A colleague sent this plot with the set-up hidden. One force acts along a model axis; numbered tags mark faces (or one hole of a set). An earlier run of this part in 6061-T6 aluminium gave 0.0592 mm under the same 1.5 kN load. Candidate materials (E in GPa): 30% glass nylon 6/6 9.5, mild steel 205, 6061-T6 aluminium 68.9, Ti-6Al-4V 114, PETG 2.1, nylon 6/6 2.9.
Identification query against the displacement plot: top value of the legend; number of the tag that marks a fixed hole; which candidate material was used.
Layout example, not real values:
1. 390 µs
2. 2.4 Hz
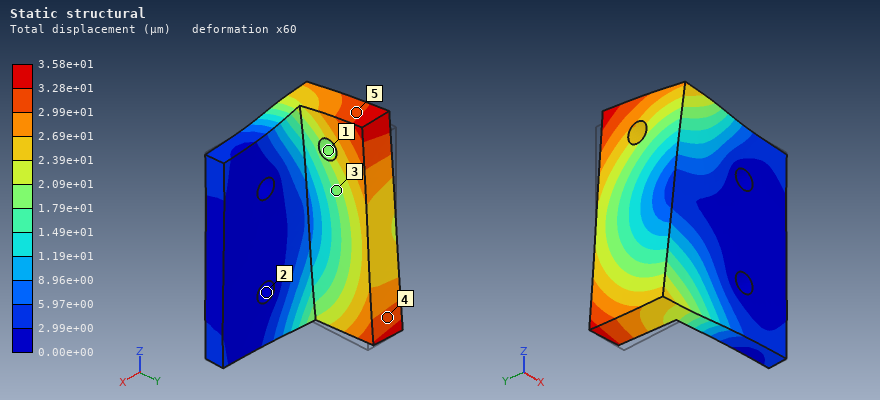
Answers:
1. 3.58e+01 µm
2. 2
3. Ti-6Al-4V
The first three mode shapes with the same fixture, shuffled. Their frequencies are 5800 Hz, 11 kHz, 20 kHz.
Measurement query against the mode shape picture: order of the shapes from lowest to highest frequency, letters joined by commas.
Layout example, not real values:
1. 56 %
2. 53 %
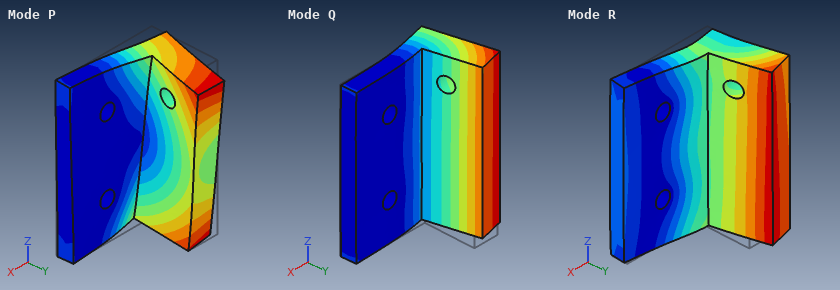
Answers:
1. Q, P, R
